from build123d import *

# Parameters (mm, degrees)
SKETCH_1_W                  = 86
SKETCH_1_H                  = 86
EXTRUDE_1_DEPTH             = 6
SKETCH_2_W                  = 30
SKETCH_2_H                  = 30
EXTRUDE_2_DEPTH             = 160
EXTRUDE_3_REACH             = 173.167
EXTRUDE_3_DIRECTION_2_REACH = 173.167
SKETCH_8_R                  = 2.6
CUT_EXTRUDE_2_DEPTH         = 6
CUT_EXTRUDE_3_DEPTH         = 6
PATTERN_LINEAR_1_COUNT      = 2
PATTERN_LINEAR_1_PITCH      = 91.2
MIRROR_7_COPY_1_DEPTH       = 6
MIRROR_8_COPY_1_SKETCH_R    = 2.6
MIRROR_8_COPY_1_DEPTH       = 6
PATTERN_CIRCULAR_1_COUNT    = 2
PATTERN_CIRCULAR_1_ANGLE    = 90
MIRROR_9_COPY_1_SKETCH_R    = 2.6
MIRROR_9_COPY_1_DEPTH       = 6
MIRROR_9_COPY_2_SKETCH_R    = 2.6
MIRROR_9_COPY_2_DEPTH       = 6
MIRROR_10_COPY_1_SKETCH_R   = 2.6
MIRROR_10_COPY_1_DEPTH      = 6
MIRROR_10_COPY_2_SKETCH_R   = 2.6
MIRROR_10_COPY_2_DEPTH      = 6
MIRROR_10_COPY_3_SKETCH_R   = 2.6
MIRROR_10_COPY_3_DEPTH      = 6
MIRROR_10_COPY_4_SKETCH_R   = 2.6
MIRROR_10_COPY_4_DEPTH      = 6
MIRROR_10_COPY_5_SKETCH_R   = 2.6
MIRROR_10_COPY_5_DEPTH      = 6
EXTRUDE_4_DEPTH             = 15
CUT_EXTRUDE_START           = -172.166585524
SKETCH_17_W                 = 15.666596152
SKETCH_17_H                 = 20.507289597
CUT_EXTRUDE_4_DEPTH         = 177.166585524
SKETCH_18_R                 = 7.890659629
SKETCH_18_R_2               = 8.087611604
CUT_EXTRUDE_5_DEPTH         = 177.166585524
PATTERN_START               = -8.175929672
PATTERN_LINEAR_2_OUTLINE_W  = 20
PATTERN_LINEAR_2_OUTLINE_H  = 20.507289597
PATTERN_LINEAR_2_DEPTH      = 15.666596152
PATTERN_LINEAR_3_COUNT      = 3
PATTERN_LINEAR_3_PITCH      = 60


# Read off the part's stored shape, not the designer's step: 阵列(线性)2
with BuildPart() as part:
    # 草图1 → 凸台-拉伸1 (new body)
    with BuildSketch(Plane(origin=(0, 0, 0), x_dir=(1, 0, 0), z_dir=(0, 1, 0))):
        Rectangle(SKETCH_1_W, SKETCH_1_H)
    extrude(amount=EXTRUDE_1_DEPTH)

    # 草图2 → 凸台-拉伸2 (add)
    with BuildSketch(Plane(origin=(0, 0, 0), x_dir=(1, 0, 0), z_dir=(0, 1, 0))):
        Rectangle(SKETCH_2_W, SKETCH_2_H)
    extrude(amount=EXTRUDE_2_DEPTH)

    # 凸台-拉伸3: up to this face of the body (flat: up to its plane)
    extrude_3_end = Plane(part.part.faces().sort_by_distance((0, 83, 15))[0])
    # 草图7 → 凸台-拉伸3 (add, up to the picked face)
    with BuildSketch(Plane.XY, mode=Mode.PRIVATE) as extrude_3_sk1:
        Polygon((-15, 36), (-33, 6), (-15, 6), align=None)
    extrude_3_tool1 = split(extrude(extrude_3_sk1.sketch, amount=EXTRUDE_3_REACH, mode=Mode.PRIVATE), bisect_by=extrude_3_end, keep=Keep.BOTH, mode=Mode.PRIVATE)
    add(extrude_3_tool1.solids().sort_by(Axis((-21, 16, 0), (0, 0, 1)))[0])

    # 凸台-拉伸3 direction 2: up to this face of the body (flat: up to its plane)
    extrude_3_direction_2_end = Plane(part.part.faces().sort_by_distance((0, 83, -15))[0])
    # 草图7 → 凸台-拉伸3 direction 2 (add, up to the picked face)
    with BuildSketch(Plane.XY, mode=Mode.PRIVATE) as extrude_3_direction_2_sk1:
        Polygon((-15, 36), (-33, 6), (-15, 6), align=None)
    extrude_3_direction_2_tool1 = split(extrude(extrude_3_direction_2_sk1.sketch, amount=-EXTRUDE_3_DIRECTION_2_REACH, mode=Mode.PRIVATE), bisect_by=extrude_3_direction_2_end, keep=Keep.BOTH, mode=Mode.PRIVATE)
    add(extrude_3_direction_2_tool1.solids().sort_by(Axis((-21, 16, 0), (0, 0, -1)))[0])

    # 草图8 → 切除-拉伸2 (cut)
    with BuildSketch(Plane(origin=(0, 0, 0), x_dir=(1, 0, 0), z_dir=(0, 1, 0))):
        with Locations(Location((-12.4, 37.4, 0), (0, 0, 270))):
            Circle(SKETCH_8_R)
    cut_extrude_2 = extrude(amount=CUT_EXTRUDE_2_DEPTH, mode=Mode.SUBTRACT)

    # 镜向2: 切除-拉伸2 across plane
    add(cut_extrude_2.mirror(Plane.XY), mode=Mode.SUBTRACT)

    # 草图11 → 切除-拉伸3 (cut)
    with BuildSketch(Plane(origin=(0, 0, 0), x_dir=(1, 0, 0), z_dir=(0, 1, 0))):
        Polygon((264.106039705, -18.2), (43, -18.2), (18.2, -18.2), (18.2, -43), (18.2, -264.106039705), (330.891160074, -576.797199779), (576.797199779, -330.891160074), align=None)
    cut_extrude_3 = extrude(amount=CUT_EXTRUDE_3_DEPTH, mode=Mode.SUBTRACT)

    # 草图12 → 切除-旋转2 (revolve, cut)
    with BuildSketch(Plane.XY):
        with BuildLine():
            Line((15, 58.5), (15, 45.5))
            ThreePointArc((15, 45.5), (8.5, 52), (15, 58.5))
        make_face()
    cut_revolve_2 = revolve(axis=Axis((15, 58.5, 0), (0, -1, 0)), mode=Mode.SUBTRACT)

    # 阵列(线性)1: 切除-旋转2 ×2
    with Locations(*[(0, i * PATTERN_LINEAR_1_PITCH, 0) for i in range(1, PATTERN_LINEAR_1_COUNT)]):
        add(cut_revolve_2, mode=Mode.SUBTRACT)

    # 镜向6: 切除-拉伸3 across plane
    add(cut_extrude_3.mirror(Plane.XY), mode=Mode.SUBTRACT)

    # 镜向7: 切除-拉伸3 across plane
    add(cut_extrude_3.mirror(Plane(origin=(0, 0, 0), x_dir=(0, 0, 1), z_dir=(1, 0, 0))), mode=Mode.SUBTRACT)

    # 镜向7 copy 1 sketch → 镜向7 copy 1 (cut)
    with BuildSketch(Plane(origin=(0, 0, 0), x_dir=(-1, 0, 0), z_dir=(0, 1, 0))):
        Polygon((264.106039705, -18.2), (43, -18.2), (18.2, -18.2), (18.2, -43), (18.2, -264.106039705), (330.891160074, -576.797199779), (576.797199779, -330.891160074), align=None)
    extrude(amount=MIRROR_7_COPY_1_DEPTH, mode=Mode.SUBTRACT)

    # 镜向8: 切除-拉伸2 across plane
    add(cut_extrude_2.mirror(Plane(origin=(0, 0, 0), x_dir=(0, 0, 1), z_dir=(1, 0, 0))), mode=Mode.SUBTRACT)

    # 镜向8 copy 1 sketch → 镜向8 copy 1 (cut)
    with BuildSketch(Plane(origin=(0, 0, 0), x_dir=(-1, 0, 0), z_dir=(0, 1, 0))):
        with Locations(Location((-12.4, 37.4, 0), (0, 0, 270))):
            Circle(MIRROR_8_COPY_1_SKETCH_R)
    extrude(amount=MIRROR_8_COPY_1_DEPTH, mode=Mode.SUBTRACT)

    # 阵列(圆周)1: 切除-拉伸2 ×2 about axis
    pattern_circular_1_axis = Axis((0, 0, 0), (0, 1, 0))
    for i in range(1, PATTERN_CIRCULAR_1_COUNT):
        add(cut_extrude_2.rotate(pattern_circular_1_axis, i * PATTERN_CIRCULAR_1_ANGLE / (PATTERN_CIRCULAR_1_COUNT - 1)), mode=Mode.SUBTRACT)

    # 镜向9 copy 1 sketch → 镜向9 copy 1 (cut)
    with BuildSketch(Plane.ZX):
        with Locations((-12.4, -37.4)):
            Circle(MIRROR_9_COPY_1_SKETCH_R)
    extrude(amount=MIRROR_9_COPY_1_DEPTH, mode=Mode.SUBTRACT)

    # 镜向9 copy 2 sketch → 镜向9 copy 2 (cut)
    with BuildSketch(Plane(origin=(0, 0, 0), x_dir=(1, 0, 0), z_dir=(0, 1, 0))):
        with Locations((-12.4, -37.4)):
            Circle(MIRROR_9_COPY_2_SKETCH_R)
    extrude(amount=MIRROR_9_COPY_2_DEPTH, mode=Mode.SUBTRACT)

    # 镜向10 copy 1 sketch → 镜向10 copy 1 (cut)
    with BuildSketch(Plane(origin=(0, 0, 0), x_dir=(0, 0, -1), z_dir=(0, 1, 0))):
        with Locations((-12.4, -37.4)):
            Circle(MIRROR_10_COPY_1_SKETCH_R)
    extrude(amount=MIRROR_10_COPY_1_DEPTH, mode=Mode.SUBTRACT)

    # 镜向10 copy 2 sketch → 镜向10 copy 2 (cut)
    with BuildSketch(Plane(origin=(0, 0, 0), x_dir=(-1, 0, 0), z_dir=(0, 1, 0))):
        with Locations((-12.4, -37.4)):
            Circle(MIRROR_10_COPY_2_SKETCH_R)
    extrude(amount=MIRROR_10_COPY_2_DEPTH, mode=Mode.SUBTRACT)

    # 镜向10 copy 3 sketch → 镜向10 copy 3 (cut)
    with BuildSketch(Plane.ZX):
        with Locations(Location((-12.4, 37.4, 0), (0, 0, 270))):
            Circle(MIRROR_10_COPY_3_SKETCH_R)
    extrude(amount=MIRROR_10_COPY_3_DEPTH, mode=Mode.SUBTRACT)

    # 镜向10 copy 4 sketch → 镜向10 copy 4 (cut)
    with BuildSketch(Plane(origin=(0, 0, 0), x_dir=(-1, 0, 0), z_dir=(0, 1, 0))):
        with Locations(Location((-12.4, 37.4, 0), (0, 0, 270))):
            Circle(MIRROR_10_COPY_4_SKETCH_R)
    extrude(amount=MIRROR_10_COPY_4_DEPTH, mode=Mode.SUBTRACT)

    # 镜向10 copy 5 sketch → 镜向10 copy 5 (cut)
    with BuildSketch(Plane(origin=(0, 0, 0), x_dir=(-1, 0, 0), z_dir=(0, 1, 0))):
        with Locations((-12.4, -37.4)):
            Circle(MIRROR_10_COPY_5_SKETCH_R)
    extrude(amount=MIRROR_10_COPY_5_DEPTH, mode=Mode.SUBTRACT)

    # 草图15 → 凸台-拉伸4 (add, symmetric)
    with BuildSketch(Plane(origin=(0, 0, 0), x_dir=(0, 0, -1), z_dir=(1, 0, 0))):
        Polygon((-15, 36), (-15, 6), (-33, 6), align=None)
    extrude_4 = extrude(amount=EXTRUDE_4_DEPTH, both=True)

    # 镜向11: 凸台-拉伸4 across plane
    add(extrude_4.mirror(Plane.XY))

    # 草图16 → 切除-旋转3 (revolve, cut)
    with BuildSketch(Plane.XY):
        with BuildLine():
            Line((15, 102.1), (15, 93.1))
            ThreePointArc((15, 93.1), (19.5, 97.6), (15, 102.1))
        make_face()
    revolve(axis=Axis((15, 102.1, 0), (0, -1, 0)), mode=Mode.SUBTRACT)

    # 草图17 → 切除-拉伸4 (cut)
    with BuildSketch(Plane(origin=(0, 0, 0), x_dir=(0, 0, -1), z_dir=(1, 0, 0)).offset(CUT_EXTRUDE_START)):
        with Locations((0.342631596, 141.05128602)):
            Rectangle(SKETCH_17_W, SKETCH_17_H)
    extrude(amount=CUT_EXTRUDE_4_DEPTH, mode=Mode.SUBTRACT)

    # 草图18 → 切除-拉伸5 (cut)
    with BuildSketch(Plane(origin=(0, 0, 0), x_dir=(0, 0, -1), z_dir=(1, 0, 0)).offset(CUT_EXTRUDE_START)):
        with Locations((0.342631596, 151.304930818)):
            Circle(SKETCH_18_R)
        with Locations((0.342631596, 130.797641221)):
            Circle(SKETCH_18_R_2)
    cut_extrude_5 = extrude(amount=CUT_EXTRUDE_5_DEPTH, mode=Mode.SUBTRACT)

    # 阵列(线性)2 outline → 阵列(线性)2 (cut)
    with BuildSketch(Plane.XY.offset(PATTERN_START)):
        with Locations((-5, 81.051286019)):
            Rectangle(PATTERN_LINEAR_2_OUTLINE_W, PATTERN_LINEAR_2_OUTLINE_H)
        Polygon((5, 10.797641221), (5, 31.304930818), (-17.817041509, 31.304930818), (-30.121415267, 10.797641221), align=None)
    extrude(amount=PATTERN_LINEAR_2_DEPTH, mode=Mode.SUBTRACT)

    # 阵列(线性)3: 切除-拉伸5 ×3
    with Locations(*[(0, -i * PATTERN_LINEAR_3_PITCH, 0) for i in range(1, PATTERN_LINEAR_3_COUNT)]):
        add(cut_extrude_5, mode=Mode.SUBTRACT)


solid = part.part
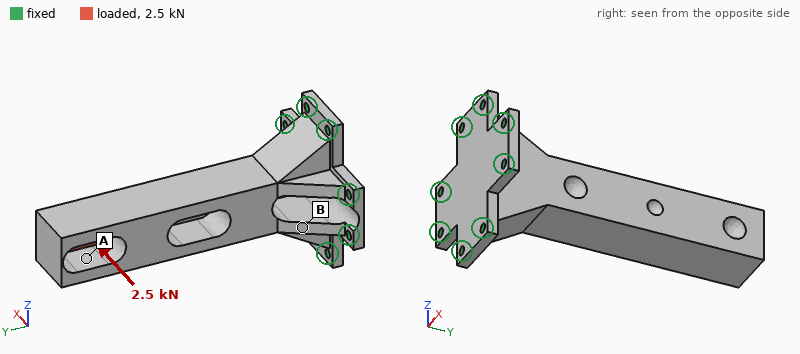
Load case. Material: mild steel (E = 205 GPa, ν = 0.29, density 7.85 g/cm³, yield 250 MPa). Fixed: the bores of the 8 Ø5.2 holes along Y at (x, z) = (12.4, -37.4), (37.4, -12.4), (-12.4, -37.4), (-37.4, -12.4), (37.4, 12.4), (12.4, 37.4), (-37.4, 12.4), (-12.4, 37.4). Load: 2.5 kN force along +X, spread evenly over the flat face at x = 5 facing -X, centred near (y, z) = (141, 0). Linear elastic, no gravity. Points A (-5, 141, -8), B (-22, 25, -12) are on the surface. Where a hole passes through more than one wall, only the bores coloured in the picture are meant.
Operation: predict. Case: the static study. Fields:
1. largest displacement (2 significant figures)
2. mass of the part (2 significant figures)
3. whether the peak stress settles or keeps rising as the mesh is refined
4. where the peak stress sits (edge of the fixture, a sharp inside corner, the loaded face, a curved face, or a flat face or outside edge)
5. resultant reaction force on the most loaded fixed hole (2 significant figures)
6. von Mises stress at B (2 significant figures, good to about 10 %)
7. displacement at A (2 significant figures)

0.26 mm
1.2 kg
keeps rising
edge of the fixture
3.7 kN
65 MPa
0.21 mm
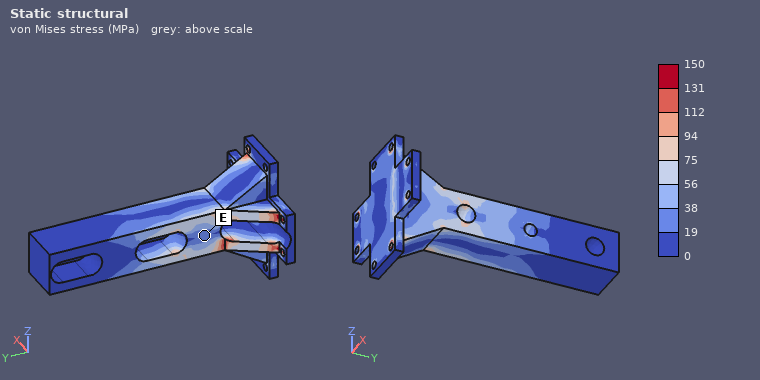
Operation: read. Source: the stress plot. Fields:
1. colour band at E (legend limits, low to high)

19 to 38 MPa
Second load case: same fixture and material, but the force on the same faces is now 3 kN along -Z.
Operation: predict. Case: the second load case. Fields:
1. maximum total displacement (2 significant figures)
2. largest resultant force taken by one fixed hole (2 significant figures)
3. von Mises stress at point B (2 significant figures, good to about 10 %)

0.22 mm
3.1 kN
30 MPa
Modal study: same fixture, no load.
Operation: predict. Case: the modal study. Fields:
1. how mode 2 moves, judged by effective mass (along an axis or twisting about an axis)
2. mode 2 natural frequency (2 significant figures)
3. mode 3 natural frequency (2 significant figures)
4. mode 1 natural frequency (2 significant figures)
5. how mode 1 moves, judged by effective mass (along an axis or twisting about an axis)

along Z
1200 Hz
4100 Hz
990 Hz
along X
